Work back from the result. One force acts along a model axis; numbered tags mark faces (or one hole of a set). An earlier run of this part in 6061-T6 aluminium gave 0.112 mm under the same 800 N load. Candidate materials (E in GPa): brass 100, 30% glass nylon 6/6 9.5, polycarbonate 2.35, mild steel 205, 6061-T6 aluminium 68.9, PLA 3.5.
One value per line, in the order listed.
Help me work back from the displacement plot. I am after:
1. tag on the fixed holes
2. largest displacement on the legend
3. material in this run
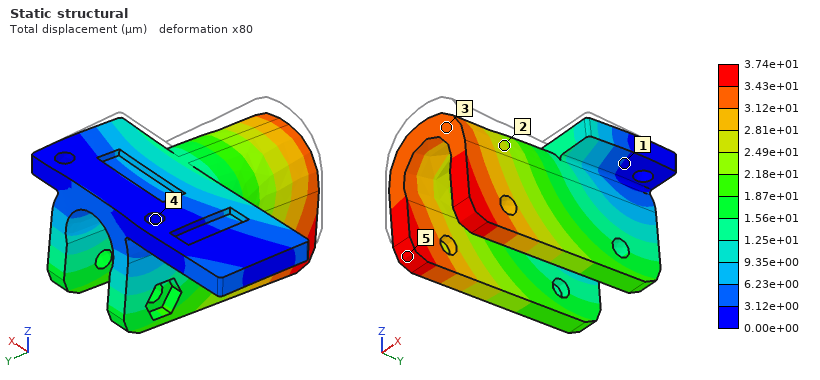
4
3.74e+01 µm
mild steel
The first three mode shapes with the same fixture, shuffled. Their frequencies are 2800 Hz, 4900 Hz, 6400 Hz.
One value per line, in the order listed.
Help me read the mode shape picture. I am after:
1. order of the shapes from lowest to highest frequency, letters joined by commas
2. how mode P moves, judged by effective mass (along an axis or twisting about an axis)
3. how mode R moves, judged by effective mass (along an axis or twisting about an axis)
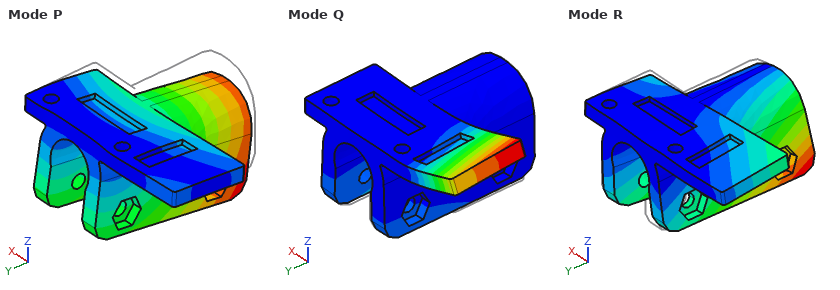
P, R, Q
along Z
along X
